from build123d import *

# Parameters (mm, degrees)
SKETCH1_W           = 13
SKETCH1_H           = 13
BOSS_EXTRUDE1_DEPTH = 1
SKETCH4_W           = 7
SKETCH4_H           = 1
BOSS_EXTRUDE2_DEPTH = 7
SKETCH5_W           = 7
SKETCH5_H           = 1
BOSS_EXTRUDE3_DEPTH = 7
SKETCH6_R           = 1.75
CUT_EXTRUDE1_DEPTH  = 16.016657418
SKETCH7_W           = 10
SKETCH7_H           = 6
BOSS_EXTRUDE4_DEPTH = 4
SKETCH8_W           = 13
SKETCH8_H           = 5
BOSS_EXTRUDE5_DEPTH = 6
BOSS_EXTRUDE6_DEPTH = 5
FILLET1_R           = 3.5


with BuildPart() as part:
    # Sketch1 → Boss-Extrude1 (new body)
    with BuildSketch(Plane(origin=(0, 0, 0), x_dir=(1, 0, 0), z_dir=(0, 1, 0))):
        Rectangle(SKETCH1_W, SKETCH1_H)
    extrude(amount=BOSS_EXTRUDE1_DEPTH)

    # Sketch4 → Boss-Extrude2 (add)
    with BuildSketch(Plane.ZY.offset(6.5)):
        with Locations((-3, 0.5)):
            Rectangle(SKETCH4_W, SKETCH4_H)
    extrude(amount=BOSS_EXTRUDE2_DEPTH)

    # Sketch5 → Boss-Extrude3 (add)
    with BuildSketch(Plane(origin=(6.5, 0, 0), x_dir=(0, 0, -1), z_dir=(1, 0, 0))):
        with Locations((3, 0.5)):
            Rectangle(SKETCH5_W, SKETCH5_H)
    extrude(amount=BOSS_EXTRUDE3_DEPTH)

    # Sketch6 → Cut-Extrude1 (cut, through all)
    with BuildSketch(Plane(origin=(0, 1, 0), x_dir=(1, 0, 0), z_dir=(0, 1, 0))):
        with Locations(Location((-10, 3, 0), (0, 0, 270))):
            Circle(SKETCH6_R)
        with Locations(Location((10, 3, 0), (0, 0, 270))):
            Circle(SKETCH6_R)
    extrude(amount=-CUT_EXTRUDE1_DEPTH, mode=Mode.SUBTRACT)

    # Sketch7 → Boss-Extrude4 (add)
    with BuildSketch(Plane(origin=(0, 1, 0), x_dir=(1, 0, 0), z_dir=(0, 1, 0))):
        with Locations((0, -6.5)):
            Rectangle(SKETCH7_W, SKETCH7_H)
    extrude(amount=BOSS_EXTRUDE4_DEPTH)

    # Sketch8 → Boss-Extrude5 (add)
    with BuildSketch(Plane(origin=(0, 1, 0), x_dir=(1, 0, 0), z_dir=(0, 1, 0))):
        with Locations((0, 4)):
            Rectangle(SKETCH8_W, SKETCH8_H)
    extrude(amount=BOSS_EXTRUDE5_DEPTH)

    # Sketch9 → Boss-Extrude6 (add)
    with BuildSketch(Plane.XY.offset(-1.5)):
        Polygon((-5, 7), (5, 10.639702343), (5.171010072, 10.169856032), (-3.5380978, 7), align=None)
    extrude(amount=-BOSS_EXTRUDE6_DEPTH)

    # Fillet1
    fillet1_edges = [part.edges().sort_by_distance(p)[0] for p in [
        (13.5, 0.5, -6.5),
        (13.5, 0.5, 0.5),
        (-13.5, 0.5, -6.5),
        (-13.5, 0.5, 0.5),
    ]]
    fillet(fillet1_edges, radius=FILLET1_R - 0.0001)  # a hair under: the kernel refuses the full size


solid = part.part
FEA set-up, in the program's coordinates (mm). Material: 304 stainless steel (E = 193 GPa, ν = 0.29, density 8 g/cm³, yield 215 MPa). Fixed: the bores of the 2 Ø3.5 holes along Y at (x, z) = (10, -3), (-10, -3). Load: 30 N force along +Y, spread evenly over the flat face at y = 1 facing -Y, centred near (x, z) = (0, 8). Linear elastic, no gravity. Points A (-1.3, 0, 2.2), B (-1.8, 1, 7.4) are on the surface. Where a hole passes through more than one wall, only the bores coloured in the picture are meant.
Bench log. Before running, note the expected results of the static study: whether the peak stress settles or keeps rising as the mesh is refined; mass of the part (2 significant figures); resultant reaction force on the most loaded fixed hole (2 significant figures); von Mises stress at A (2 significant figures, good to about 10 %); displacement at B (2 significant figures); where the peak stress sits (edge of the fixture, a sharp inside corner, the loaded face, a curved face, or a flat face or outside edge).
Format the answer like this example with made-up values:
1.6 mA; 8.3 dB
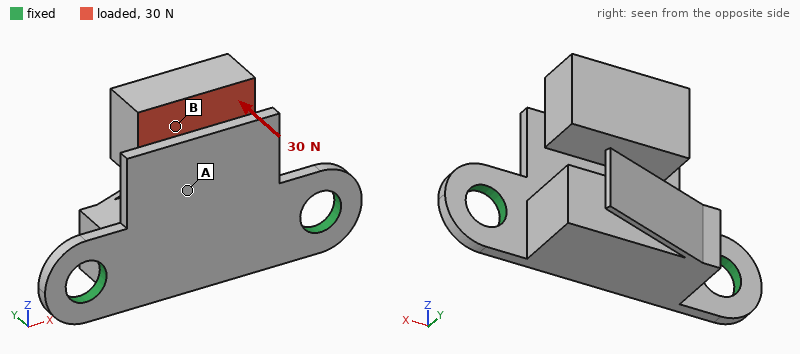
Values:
keeps rising; 7.1 g; 17 N; 70 MPa; 48 µm; a sharp inside corner
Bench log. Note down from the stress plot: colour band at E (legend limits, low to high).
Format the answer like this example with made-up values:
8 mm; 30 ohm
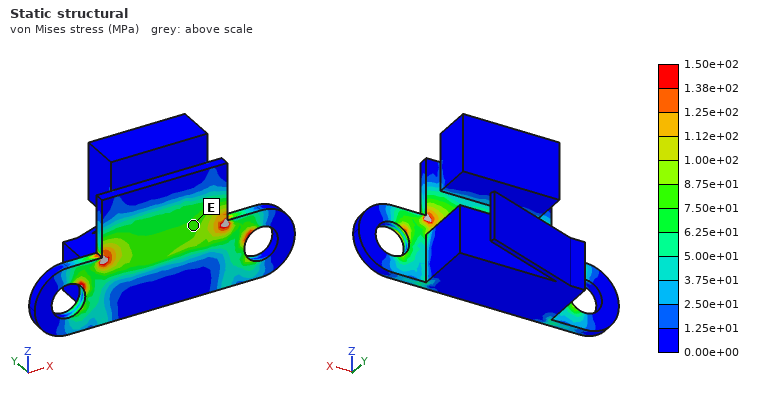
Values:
7.50e+01 to 8.75e+01 MPa
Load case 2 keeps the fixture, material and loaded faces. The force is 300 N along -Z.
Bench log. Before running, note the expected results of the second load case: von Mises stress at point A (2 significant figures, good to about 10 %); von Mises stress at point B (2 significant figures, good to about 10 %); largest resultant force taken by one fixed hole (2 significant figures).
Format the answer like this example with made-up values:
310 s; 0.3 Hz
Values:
44 MPa; 29 MPa; 150 N
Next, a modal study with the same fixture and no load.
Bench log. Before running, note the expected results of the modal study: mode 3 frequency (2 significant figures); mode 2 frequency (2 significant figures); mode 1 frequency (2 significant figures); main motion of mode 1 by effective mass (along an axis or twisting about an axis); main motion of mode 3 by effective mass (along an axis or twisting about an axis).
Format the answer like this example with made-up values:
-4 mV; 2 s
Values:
9700 Hz; 4400 Hz; 2900 Hz; along Y; along Z
